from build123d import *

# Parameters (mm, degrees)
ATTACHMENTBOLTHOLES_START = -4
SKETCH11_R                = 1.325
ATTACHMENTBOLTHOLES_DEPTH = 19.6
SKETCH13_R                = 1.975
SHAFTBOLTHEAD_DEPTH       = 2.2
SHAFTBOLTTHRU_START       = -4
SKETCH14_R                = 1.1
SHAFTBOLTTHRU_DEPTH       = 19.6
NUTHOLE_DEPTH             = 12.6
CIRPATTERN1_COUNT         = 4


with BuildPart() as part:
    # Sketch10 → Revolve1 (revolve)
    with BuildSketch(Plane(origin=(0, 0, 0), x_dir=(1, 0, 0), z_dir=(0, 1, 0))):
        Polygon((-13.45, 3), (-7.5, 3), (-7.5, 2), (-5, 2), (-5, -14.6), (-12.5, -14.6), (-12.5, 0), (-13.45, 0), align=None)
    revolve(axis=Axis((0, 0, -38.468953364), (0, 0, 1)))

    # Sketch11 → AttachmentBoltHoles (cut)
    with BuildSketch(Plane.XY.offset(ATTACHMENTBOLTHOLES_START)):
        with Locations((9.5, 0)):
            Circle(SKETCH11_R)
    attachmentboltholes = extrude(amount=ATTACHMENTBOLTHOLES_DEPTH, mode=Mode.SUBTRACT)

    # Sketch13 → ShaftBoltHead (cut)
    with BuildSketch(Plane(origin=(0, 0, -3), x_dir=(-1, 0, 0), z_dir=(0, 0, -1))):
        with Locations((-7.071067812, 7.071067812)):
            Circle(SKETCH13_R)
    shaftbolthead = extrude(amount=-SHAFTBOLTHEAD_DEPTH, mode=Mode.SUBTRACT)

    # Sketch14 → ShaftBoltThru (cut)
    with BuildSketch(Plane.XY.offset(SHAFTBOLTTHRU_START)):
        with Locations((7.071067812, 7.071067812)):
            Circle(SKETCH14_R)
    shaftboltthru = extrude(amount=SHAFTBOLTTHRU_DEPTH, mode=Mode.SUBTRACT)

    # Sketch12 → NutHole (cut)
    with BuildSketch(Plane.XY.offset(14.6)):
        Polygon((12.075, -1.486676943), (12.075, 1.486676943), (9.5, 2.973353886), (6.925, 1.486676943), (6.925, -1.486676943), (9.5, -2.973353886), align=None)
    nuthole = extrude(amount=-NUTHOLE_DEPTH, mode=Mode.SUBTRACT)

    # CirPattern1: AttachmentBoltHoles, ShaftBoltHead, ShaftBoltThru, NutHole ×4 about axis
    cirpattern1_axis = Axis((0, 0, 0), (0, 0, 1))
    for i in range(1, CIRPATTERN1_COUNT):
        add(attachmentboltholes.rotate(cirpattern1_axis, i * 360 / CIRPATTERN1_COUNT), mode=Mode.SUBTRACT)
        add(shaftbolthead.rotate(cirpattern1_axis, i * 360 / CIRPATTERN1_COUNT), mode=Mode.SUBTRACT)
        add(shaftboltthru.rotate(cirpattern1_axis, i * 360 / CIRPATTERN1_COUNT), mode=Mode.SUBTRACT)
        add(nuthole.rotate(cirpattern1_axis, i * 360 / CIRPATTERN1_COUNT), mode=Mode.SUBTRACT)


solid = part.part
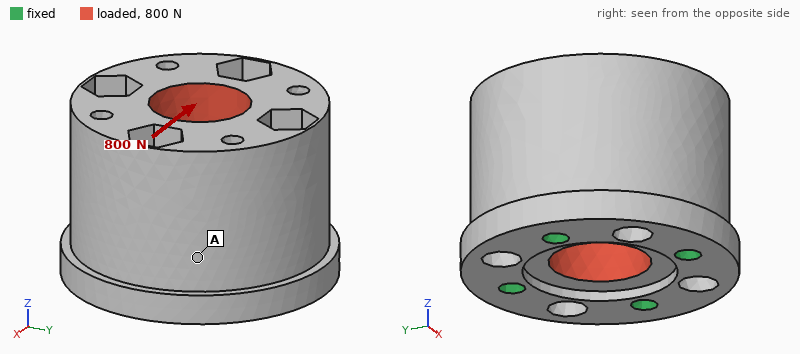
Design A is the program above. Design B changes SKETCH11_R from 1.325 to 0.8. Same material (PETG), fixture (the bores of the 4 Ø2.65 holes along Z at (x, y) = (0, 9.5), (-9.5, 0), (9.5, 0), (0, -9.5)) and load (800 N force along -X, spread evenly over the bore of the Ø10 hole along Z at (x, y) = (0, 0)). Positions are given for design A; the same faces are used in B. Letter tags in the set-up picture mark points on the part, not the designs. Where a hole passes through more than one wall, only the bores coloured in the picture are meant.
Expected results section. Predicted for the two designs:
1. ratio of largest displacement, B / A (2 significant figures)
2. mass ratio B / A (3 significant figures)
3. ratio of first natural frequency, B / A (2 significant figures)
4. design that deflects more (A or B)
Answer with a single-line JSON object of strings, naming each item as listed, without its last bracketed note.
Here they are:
{"ratio of largest displacement, B / A": "1.2", "mass ratio B / A": "1.01", "ratio of first natural frequency, B / A": "0.90", "design that deflects more": "B"}
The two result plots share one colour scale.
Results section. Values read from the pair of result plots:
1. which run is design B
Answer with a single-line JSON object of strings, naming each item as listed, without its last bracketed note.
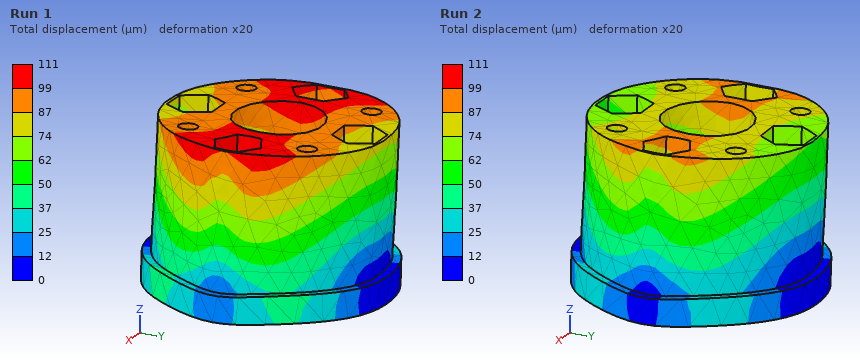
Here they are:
{"which run is design B": "Run 1"}
